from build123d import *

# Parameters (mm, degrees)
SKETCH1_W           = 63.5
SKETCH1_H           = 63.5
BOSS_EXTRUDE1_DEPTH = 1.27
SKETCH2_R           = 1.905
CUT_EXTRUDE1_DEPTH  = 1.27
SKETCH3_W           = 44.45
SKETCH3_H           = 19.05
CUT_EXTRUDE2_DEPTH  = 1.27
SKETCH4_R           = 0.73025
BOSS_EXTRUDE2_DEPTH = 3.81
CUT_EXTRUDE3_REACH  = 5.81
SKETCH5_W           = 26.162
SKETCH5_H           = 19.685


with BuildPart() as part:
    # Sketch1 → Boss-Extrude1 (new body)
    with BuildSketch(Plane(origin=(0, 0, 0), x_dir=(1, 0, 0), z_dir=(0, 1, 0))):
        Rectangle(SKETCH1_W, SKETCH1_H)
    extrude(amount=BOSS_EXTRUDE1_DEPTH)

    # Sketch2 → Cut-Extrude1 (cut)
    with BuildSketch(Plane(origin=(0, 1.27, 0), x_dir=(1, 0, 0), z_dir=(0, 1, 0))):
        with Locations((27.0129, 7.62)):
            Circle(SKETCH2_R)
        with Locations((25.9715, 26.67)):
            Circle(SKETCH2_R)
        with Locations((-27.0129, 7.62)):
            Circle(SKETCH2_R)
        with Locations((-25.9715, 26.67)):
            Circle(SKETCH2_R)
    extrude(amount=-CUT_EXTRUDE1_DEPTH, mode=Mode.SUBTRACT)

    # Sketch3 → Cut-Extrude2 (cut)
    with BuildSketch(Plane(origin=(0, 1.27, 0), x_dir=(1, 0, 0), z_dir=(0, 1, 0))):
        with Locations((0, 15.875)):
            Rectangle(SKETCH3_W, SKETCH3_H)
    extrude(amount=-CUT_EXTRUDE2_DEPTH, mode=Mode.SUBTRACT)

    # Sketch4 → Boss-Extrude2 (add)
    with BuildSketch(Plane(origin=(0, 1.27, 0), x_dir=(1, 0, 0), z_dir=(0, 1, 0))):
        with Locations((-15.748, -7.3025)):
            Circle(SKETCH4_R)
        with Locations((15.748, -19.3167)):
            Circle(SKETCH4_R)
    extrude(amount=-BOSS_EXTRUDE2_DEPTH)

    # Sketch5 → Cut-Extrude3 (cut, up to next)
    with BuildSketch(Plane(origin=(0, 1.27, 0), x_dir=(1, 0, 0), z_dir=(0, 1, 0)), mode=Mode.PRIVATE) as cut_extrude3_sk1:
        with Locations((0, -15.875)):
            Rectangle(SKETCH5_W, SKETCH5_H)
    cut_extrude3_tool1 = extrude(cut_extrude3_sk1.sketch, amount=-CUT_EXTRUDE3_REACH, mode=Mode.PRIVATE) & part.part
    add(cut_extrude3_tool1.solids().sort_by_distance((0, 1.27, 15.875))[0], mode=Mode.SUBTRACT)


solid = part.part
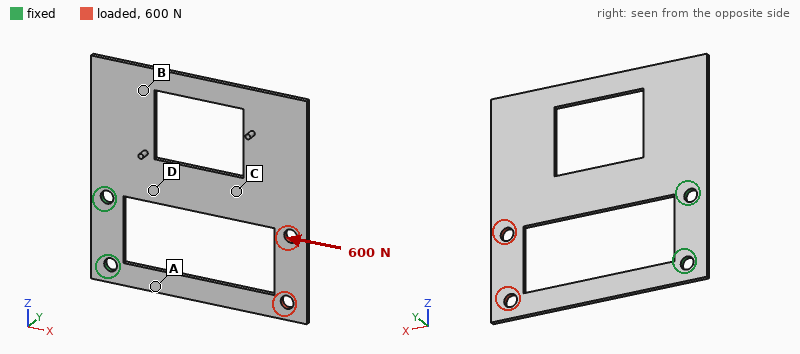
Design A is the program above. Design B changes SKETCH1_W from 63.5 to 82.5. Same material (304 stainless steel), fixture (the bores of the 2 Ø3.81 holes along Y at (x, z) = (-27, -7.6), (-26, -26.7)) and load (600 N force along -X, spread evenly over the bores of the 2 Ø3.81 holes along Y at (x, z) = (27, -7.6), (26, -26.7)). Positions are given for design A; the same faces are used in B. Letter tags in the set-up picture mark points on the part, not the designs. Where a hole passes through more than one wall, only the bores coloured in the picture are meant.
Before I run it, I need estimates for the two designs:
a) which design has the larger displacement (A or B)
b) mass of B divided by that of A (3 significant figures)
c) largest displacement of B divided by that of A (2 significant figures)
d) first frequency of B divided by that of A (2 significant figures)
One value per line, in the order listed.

A
1.46
0.90
0.76
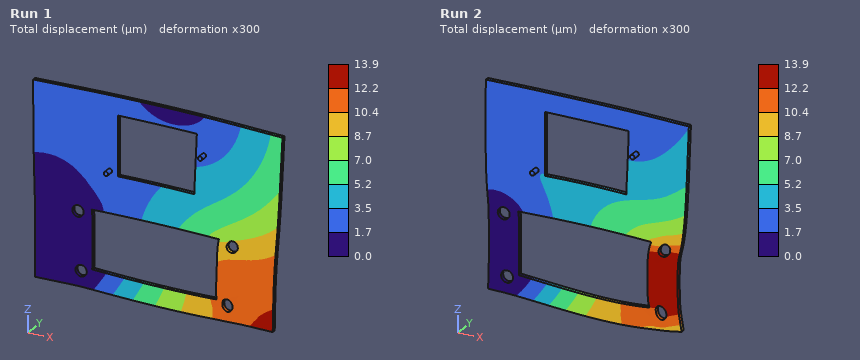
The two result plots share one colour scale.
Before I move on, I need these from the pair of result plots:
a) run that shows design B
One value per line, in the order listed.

Run 1
